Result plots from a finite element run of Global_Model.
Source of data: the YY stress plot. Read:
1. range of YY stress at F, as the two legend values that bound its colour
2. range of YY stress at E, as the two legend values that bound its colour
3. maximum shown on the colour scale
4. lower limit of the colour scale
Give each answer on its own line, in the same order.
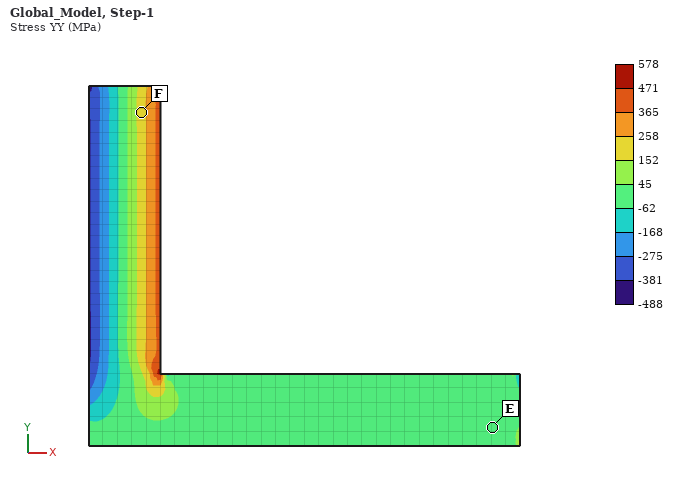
152 to 258 MPa
-62 to 45 MPa
578 MPa
-488 MPa
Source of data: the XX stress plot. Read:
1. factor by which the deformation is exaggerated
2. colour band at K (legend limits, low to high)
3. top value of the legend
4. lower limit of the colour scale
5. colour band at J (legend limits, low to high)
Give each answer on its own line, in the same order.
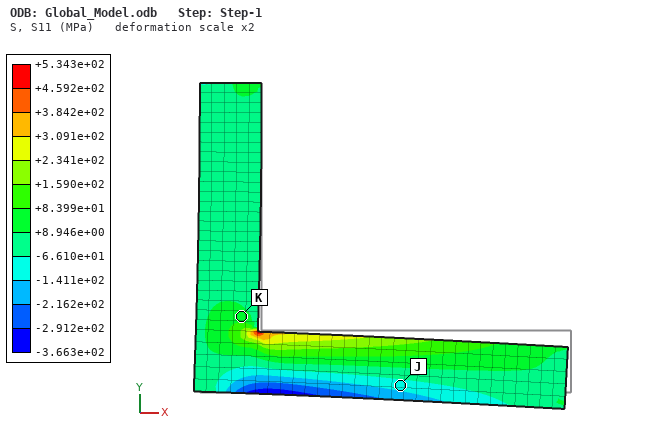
2
+8.946e+00 to +8.399e+01 MPa
+5.343e+02 MPa
-3.663e+02 MPa
-1.411e+02 to -6.610e+01 MPa
